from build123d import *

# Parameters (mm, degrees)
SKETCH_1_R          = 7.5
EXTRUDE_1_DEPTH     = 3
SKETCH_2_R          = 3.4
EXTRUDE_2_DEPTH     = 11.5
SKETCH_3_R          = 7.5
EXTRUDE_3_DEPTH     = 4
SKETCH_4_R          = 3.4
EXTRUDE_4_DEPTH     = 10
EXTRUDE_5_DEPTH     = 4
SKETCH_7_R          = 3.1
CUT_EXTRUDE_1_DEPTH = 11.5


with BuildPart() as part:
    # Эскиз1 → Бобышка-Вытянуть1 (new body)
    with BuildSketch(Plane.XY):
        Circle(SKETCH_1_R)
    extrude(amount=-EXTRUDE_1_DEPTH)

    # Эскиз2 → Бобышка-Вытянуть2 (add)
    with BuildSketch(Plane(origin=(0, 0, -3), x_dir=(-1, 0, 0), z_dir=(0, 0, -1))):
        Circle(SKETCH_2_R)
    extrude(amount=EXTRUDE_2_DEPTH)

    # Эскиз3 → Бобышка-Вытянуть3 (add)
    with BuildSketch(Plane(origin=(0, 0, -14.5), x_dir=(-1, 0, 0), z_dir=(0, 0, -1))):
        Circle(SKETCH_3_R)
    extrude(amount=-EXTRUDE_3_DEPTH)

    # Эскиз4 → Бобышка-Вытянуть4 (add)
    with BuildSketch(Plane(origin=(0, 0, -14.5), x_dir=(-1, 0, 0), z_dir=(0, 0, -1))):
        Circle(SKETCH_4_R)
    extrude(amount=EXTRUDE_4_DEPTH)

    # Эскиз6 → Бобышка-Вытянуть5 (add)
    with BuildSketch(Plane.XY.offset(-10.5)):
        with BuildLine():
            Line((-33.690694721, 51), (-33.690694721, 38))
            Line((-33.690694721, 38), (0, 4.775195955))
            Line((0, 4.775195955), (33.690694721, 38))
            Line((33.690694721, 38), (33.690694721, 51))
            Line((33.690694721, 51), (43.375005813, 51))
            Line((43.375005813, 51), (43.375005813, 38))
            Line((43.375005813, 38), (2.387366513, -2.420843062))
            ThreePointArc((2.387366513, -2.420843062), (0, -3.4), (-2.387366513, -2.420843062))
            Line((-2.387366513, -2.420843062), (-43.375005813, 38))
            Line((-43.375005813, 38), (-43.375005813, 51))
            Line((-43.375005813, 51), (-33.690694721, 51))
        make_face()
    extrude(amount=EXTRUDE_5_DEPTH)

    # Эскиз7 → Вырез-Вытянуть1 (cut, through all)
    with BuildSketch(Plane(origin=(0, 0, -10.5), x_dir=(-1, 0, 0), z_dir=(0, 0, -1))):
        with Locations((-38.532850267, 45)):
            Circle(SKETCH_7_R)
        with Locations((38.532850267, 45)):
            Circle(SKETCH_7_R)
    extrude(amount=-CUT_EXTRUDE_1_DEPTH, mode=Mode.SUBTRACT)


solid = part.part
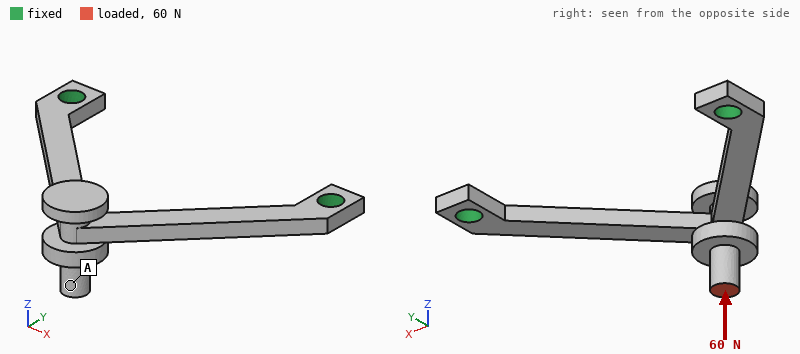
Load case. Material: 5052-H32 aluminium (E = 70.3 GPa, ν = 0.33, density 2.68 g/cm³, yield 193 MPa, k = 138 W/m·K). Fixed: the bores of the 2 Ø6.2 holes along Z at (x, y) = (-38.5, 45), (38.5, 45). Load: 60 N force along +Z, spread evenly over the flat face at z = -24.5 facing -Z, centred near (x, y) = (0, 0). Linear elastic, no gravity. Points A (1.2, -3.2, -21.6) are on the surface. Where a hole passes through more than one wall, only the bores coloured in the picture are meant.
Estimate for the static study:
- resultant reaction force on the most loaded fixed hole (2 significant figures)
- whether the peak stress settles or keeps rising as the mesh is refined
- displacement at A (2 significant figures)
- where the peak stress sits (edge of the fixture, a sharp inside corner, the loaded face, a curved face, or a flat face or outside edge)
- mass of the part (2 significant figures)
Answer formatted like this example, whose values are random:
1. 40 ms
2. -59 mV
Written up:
1. 30 N
2. keeps rising
3. 0.50 mm
4. a sharp inside corner
5. 15 g
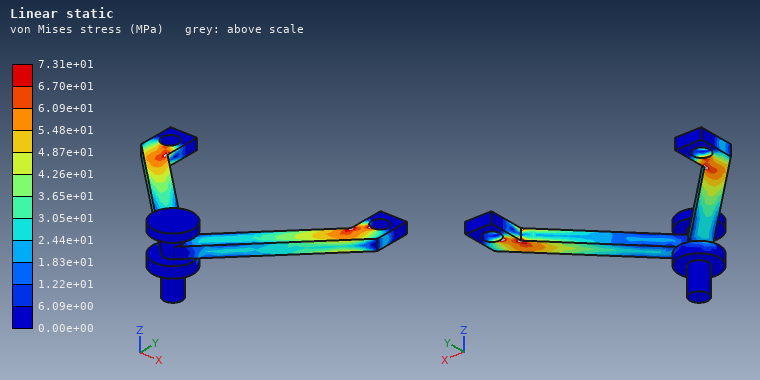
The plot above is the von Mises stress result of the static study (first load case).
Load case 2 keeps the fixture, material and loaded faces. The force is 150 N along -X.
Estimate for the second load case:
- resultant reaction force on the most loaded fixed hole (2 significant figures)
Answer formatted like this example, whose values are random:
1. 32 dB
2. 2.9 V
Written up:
1. 110 N
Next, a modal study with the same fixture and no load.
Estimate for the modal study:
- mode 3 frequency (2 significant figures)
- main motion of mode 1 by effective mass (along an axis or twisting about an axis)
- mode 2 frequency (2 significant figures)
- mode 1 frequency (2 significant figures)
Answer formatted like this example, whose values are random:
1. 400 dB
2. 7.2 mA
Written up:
1. 3700 Hz
2. along Z
3. 3600 Hz
4. 710 Hz
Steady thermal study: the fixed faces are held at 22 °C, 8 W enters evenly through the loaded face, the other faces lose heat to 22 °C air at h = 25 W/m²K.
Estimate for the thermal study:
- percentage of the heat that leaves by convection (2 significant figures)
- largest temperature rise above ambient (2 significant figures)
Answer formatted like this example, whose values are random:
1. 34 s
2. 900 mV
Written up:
1. 30 %
2. 60 K
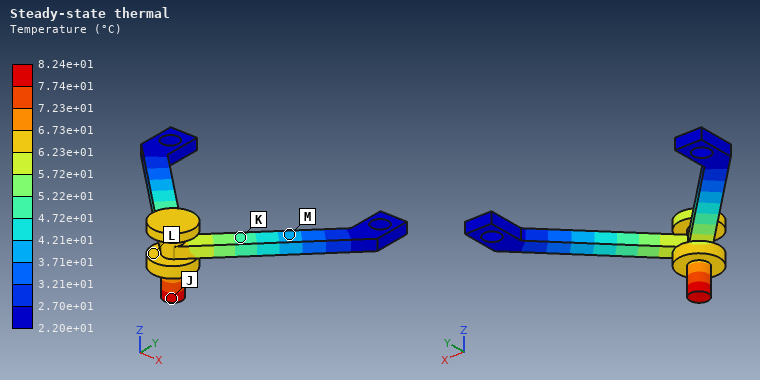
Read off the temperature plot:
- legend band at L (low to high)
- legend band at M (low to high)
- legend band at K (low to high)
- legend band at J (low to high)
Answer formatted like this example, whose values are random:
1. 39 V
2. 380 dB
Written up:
1. 6.23e+01 to 6.73e+01 °C
2. 3.71e+01 to 4.21e+01 °C
3. 4.72e+01 to 5.22e+01 °C
4. 7.74e+01 to 8.24e+01 °C
